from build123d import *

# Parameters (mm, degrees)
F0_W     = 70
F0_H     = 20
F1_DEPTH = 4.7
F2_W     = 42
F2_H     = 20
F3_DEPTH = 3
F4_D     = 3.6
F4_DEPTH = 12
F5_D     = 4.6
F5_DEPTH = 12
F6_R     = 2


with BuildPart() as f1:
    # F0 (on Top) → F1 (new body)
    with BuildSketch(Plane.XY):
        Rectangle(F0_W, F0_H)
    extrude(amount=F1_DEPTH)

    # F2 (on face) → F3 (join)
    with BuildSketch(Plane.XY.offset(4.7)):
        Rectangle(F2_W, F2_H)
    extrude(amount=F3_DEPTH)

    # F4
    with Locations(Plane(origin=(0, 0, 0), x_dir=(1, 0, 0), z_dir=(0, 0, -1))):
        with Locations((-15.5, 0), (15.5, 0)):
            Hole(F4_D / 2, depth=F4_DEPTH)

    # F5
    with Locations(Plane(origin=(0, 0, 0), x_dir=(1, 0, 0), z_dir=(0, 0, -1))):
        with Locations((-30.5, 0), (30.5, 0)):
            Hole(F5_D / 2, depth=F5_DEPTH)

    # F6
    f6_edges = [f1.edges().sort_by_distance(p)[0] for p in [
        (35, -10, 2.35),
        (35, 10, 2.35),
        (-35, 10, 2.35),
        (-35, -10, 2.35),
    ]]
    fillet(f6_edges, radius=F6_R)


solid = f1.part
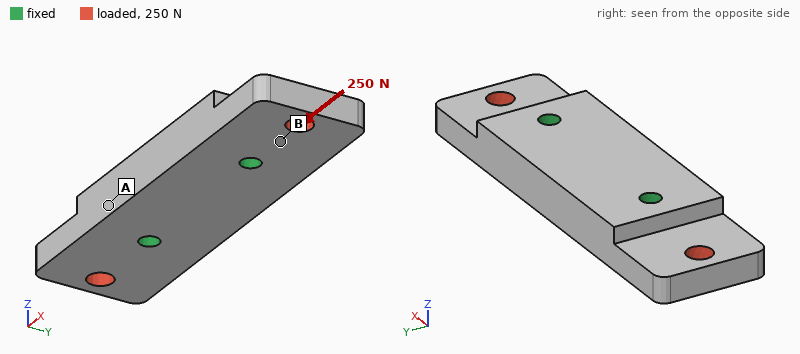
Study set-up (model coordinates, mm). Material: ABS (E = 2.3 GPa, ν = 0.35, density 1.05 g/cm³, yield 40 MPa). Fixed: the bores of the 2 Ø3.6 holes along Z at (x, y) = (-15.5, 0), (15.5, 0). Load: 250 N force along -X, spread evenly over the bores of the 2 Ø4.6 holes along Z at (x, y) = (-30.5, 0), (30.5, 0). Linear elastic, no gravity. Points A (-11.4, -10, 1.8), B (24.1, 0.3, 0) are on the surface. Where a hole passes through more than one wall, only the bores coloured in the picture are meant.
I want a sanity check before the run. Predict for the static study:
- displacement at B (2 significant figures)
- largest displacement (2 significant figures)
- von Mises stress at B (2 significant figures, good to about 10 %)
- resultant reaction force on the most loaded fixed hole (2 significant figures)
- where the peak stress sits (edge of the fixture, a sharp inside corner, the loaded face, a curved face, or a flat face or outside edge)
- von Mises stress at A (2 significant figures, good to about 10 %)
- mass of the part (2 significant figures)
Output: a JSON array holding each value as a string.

["9.4 µm", "25 µm", "2.4 MPa", "130 N", "the loaded face", "0.63 MPa", "9.2 g"]
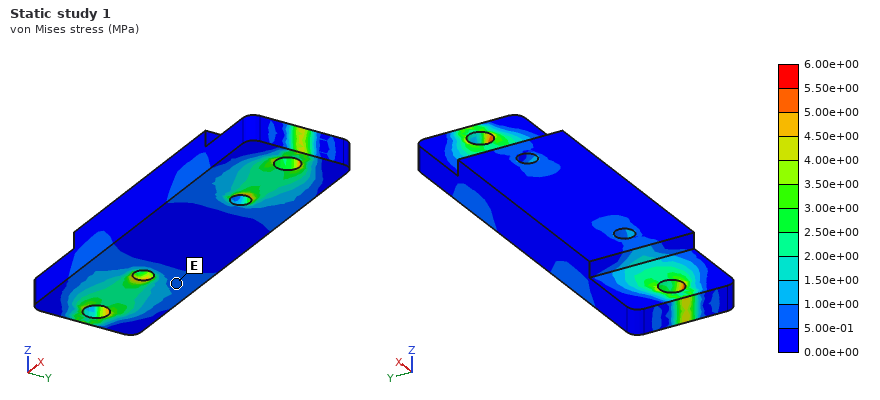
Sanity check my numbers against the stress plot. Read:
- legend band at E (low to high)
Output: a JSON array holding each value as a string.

["5.00e-01 to 1.00e+00 MPa"]
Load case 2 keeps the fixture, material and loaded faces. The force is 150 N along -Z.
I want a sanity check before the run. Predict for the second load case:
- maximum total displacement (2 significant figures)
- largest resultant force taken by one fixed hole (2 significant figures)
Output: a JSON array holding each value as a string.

["0.22 mm", "75 N"]
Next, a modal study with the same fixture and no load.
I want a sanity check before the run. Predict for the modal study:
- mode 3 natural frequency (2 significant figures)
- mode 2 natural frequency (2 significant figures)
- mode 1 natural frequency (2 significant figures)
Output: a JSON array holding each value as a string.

["6200 Hz", "3900 Hz", "3800 Hz"]
